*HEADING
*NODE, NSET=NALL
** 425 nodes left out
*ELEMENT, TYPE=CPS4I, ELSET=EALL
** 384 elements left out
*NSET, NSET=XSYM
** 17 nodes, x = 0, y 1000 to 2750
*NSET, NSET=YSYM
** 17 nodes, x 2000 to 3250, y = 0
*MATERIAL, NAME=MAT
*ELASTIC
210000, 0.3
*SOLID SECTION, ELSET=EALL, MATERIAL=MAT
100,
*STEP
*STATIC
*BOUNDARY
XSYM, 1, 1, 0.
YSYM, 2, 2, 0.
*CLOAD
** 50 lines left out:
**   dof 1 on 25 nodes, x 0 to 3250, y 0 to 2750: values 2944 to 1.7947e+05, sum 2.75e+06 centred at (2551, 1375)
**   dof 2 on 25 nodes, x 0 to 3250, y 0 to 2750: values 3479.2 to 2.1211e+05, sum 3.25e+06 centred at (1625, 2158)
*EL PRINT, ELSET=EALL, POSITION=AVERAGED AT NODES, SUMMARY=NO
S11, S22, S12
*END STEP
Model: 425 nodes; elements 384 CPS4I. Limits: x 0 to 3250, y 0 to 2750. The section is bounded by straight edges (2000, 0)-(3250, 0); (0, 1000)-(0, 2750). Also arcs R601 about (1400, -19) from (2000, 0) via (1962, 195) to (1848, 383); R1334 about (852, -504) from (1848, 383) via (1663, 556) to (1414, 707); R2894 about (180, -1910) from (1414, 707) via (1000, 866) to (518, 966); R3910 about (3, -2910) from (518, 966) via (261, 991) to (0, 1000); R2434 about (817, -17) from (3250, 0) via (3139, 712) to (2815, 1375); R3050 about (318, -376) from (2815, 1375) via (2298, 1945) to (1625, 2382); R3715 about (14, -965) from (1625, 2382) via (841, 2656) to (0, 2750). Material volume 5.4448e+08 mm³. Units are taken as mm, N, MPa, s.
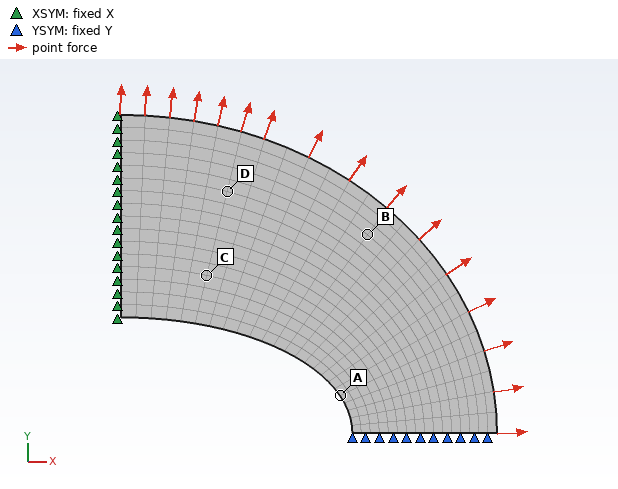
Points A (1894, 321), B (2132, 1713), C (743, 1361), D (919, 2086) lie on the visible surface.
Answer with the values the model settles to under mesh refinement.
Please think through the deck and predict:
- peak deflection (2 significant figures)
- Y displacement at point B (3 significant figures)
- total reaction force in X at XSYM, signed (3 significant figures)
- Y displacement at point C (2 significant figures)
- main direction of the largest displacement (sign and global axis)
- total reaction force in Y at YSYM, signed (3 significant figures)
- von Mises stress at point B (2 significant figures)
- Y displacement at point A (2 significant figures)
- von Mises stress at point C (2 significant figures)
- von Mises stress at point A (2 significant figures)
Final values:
0.56 mm
0.225 mm
-2.75e+06 N
0.50 mm
+Y
-3.25e+06 N
18 MPa
0.15 mm
10 MPa
63 MPa
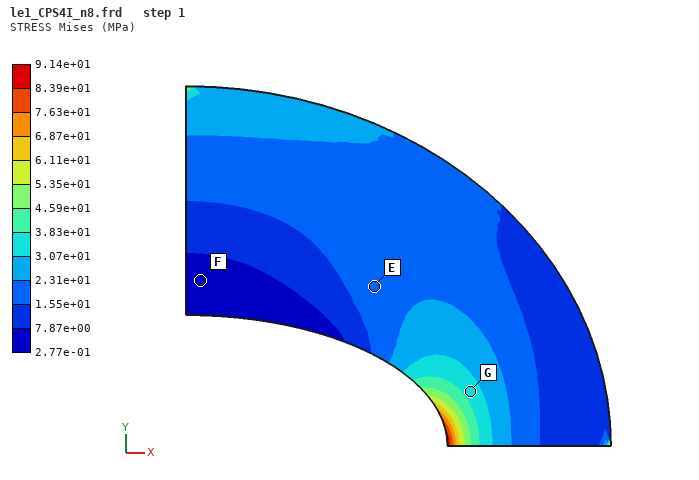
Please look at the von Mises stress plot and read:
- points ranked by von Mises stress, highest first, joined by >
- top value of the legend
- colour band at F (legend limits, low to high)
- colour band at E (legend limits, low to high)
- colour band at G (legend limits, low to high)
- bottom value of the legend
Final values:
G > E > F
9.14e+01 MPa
2.77e-01 to 7.87e+00 MPa
1.55e+01 to 2.31e+01 MPa
3.07e+01 to 3.83e+01 MPa
2.77e-01 MPa
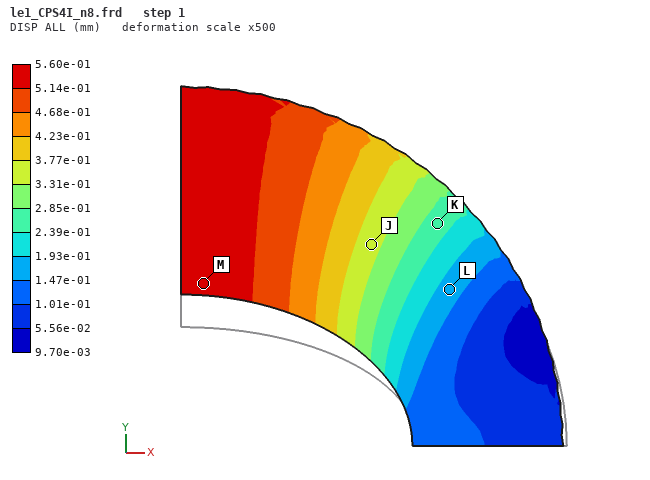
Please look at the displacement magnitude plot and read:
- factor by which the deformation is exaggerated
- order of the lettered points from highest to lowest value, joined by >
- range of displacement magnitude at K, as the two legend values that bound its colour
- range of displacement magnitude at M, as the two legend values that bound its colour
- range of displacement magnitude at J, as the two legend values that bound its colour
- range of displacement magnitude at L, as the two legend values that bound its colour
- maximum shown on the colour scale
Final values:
500
M > J > K > L
2.39e-01 to 2.85e-01 mm
5.14e-01 to 5.60e-01 mm
3.31e-01 to 3.77e-01 mm
1.47e-01 to 1.93e-01 mm
5.60e-01 mm
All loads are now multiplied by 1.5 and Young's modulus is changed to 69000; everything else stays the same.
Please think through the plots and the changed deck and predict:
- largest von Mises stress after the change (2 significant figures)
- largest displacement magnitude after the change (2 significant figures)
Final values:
140 MPa
2.6 mm
